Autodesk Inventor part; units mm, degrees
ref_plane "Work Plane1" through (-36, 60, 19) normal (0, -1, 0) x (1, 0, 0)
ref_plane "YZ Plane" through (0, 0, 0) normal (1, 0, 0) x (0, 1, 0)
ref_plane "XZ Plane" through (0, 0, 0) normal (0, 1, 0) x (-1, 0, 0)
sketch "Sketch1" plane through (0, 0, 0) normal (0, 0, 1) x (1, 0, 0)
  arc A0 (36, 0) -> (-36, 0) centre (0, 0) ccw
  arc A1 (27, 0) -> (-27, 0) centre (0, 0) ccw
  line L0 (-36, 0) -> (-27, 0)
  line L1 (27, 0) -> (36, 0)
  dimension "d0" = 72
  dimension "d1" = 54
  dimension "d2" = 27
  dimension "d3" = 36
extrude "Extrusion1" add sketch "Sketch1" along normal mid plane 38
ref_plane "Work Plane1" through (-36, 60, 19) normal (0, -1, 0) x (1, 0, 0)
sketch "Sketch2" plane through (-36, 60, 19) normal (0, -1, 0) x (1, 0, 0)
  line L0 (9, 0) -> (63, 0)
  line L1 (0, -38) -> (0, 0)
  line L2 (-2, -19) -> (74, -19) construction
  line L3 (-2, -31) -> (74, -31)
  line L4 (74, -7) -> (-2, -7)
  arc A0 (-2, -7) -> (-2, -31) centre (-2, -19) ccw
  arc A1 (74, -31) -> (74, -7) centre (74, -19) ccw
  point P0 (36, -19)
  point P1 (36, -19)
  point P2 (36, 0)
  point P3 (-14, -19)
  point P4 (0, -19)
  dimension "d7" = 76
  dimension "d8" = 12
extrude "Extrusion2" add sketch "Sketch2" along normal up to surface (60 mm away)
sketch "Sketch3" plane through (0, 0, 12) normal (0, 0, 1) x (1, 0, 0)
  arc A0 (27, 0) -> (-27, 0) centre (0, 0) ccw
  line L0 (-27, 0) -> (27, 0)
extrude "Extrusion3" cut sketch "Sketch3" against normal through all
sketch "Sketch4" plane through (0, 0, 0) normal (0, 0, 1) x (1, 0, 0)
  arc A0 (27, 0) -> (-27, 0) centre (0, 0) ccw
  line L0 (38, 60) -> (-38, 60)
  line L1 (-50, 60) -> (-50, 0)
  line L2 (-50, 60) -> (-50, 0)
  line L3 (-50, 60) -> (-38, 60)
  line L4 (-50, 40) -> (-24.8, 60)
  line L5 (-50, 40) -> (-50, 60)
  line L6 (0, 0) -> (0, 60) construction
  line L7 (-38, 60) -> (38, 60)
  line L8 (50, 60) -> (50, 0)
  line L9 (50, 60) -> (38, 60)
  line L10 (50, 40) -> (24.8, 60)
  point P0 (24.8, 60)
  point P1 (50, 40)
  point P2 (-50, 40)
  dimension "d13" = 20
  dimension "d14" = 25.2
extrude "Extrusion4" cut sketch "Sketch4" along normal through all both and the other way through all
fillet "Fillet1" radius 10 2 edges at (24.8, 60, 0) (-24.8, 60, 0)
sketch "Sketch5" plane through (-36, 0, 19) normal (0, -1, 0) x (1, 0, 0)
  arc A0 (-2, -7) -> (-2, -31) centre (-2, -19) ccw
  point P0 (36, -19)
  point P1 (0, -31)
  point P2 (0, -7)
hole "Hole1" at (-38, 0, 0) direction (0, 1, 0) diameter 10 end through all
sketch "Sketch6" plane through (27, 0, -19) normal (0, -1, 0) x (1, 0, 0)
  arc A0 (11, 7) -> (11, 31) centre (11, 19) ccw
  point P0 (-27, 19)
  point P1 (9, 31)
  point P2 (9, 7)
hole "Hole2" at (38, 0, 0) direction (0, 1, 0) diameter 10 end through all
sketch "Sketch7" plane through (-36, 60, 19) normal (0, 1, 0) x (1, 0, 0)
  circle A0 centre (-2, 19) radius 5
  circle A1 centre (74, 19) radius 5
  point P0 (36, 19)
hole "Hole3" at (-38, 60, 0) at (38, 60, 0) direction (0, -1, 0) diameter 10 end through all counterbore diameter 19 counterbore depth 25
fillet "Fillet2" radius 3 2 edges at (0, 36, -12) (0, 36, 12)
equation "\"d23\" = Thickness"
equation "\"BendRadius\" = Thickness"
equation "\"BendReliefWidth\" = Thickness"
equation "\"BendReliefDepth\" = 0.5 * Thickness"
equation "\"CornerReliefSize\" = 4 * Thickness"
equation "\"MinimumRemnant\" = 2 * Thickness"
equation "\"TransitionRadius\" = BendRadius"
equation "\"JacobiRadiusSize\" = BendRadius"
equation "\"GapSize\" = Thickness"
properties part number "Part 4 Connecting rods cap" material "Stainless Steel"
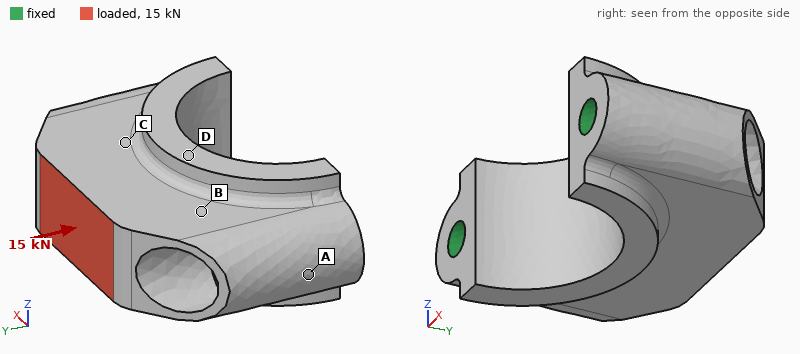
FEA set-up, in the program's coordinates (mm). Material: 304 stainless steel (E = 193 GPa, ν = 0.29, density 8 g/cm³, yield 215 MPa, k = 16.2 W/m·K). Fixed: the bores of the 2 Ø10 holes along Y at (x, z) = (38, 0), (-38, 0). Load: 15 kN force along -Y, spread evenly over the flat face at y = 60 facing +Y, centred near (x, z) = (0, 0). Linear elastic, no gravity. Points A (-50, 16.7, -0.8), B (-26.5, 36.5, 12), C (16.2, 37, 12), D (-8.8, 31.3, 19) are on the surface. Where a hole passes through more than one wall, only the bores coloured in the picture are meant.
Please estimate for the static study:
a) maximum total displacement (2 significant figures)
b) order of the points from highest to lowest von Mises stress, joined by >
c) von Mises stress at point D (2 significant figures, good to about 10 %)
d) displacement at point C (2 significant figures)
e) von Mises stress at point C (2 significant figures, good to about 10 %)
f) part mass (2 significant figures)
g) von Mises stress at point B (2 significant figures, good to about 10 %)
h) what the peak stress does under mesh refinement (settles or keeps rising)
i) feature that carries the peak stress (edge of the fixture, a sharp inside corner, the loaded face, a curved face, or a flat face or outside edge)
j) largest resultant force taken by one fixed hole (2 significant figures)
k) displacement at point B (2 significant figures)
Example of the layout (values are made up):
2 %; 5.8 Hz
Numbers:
5.1 µm; C > B > D > A; 6.4 MPa; 2.9 µm; 17 MPa; 790 g; 14 MPa; keeps rising; edge of the fixture; 8.8 kN; 1.8 µm
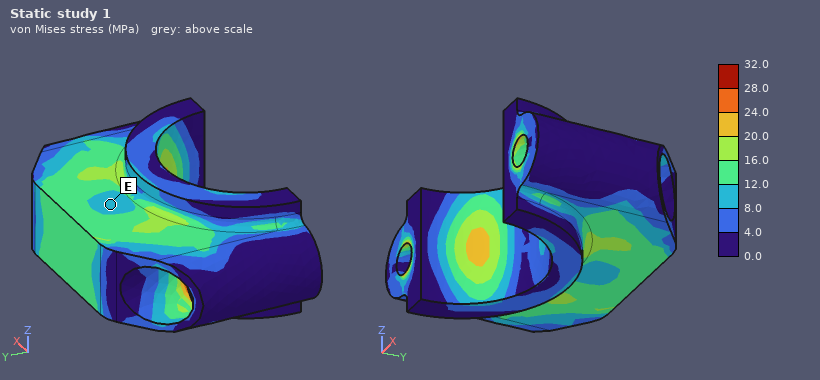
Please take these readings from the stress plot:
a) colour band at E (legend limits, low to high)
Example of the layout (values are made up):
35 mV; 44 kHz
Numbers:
8.0 to 12.0 MPa
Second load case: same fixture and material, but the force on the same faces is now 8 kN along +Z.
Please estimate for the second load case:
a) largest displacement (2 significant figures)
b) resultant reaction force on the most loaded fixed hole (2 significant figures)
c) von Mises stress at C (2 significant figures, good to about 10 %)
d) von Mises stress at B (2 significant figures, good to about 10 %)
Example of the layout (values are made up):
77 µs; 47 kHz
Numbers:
25 µm; 4.0 kN; 38 MPa; 37 MPa
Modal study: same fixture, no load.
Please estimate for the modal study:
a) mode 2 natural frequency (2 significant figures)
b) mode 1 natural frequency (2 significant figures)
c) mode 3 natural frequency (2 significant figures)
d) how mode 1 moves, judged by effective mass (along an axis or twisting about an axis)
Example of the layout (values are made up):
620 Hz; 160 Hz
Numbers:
16 kHz; 7700 Hz; 16 kHz; along Z
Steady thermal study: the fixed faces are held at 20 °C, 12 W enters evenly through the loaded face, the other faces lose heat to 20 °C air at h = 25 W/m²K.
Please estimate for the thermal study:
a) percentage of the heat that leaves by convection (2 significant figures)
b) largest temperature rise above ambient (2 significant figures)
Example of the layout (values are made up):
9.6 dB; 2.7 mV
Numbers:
21 %; 23 K
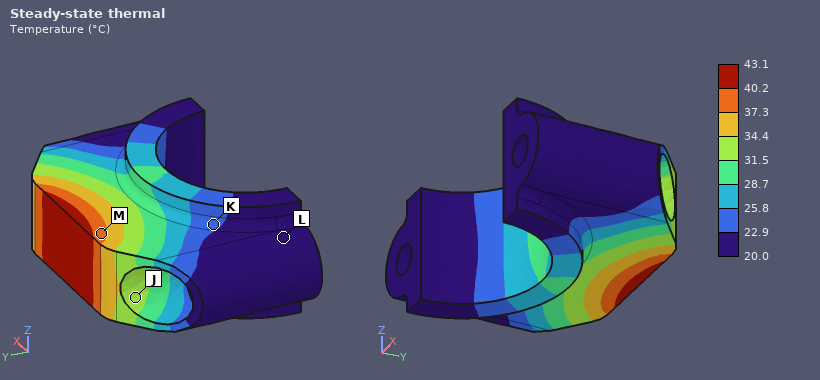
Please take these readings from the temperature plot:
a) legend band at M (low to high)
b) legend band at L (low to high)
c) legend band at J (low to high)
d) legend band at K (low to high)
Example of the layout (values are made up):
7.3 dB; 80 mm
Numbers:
37.3 to 40.2 °C; 20.0 to 22.9 °C; 31.5 to 34.4 °C; 22.9 to 25.8 °C
